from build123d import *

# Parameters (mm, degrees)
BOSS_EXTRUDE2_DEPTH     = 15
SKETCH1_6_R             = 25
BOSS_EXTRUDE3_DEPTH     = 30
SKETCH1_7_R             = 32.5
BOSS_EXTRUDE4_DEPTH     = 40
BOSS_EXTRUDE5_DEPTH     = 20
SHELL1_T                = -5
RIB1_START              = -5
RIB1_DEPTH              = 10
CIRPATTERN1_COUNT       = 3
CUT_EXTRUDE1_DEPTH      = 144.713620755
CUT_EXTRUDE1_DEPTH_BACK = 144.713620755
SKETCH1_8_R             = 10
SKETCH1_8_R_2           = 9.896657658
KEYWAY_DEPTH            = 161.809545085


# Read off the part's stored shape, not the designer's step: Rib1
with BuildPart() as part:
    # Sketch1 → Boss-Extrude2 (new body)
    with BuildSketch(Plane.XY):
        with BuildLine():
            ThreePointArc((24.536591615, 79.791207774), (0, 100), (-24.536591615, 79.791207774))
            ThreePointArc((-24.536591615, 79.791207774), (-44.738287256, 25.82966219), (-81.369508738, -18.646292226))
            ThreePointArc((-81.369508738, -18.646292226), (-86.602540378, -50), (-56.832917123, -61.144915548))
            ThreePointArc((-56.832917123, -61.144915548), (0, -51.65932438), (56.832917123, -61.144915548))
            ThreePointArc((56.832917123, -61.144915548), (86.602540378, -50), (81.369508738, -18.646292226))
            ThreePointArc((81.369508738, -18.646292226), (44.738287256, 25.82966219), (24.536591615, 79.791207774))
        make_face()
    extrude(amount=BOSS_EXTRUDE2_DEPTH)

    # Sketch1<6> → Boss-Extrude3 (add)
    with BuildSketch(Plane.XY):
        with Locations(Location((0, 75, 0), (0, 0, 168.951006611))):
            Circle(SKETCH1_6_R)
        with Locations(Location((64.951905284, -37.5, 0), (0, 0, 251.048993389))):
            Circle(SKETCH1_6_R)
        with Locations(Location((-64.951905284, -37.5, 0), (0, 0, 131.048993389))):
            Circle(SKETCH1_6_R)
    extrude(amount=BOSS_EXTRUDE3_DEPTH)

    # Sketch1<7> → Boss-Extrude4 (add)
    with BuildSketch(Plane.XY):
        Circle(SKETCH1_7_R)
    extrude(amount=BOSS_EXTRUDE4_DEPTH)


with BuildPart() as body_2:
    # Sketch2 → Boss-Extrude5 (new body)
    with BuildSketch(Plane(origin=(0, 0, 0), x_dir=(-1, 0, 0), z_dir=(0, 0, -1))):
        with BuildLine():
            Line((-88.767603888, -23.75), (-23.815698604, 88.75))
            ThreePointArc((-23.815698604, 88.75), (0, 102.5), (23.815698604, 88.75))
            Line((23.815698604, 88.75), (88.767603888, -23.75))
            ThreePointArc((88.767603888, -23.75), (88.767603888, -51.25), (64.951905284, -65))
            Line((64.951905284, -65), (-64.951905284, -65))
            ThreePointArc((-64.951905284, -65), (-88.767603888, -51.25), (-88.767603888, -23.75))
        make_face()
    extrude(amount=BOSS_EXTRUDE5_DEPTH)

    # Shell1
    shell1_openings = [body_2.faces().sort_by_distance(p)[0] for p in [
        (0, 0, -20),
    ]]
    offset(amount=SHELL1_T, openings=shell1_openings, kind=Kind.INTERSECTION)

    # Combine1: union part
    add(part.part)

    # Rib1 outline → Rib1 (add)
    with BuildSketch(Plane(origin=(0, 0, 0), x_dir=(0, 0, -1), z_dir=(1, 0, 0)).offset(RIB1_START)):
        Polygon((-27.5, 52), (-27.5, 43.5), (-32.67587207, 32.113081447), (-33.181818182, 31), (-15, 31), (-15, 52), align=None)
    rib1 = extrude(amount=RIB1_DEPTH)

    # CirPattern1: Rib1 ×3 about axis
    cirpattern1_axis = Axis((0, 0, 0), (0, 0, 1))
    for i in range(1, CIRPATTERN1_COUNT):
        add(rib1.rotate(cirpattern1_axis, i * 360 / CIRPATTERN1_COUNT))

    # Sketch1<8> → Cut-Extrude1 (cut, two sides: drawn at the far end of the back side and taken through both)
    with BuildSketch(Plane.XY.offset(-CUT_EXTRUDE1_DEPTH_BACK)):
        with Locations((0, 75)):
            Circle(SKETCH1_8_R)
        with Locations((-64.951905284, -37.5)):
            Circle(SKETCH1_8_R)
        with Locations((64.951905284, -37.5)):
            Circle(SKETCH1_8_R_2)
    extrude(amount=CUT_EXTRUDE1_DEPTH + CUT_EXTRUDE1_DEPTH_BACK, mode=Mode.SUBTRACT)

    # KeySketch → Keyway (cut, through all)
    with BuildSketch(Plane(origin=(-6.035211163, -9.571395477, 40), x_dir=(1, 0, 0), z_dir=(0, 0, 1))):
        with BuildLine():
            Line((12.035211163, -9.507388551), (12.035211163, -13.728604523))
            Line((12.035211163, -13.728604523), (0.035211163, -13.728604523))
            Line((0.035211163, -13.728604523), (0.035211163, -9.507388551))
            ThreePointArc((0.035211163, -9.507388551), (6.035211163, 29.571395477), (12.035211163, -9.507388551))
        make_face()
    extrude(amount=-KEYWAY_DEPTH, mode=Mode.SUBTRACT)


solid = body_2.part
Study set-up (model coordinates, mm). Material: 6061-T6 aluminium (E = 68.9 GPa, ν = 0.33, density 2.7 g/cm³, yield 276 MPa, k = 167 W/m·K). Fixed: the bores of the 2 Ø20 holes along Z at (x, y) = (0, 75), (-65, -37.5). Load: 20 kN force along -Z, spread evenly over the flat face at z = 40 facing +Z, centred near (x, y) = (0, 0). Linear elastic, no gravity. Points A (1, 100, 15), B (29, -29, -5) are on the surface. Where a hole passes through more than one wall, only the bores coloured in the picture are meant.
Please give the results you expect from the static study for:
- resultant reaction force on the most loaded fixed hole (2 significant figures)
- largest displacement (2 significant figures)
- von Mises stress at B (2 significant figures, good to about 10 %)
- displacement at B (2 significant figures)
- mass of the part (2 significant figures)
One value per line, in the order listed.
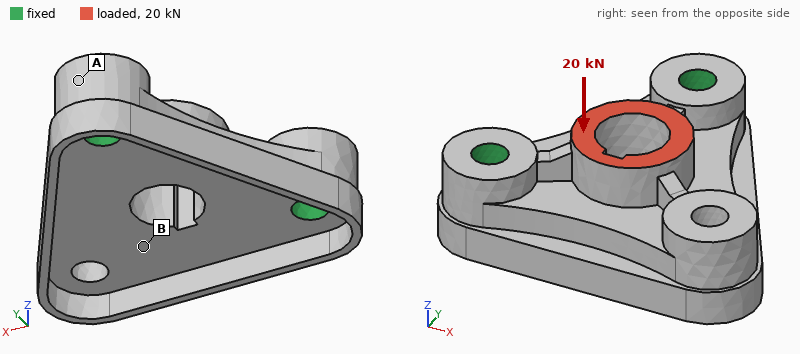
10 kN
0.25 mm
11 MPa
0.13 mm
1.3 kg
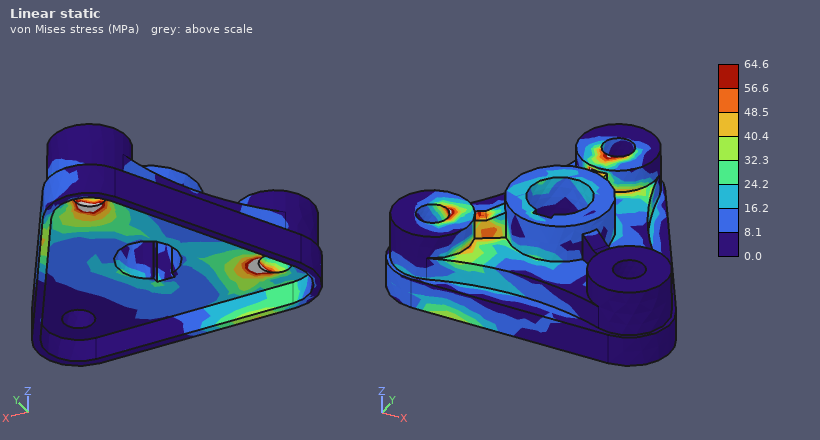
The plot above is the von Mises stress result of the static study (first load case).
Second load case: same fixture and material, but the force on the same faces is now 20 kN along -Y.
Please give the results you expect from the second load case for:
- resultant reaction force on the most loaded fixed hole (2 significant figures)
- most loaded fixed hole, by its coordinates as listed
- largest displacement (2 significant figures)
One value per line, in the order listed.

15 kN
(0, 75)
0.15 mm
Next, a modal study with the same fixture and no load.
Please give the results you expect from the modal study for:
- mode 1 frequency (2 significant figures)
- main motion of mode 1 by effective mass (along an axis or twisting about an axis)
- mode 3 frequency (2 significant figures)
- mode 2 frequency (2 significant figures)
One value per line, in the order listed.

1400 Hz
along Z
5100 Hz
4300 Hz
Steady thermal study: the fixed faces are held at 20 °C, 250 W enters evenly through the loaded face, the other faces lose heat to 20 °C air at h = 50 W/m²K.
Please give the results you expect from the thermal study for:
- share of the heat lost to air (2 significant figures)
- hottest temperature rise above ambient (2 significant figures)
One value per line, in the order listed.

21 %
40 K
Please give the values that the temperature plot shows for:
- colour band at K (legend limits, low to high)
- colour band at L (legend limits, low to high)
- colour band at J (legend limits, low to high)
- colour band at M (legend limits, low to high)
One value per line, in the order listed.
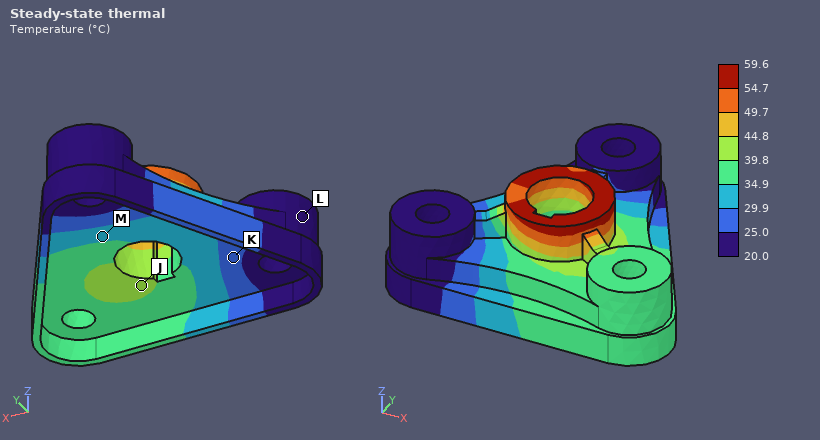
25.0 to 29.9 °C
20.0 to 25.0 °C
39.8 to 44.8 °C
29.9 to 34.9 °C
